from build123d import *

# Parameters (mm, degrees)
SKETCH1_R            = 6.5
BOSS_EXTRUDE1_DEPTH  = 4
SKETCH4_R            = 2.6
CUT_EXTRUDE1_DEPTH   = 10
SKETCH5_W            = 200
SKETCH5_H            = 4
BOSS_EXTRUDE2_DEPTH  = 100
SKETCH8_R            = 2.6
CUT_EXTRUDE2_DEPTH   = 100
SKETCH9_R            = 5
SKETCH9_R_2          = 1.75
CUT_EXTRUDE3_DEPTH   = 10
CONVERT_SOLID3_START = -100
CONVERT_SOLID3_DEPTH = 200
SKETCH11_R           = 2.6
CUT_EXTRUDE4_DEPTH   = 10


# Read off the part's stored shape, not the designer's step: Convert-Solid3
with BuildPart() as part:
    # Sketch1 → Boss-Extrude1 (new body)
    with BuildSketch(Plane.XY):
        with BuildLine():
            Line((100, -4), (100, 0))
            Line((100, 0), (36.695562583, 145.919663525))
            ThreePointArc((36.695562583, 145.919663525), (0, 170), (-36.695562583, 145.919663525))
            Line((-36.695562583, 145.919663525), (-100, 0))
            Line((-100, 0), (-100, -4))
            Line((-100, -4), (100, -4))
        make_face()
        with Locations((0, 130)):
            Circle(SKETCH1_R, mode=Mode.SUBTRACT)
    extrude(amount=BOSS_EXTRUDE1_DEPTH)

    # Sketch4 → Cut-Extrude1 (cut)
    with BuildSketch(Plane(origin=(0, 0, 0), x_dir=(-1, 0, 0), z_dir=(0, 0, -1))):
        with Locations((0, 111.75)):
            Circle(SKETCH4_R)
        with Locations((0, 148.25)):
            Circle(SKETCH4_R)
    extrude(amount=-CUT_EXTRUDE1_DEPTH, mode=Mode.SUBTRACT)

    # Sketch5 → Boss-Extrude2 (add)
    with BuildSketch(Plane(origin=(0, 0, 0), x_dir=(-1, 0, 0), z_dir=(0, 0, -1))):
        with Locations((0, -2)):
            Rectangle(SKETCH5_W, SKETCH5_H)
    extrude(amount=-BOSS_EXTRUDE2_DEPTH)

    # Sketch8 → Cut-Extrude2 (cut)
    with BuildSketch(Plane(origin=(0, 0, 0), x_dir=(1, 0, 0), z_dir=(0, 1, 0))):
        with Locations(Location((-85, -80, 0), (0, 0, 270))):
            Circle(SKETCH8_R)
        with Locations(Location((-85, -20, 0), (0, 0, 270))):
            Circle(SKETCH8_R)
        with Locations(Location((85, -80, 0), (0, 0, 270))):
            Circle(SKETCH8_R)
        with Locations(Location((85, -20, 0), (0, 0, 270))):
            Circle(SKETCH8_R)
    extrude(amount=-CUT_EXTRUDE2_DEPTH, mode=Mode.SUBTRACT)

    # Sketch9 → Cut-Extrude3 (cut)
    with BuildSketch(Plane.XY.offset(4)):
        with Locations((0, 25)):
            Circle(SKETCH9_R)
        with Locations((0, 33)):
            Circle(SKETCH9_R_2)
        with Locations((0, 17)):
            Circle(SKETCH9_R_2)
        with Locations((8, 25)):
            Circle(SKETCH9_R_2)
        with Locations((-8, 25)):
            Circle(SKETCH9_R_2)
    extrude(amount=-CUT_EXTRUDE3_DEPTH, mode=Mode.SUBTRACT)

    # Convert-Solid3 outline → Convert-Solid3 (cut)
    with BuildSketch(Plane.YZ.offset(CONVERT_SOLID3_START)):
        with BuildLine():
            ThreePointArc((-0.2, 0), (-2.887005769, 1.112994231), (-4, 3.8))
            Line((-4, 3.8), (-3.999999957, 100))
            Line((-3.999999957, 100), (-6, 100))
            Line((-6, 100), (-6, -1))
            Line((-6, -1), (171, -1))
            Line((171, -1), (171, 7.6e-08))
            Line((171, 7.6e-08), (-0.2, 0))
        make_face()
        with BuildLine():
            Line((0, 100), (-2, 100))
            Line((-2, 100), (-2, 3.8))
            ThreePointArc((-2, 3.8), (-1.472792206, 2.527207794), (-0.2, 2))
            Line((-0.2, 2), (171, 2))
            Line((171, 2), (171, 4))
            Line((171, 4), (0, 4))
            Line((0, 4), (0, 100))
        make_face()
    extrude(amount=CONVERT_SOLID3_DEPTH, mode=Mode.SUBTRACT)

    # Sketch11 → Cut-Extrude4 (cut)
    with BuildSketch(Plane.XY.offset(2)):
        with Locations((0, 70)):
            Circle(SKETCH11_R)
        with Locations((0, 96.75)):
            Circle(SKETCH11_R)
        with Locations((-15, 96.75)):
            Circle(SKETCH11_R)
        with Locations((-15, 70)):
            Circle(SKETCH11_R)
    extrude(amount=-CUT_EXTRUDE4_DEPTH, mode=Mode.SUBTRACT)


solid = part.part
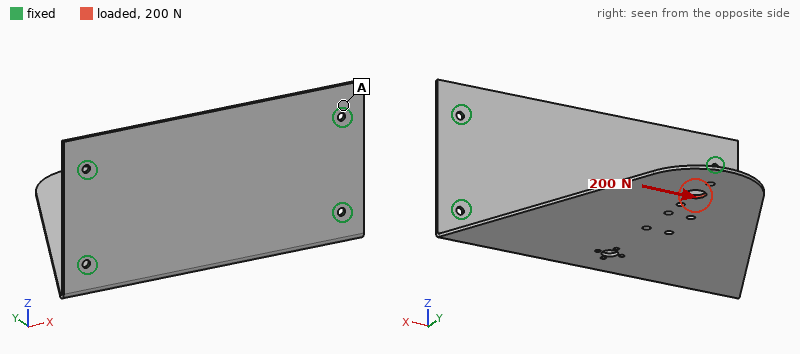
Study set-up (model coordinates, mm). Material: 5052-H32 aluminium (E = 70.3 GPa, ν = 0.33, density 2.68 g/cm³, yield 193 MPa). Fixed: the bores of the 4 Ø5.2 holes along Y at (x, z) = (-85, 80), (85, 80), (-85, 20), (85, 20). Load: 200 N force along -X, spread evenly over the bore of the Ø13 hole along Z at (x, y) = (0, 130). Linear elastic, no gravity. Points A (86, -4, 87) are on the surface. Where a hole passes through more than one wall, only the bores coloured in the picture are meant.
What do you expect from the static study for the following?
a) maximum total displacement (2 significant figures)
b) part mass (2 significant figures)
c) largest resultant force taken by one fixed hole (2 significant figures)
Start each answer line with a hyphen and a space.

- 0.37 mm
- 220 g
- 190 N
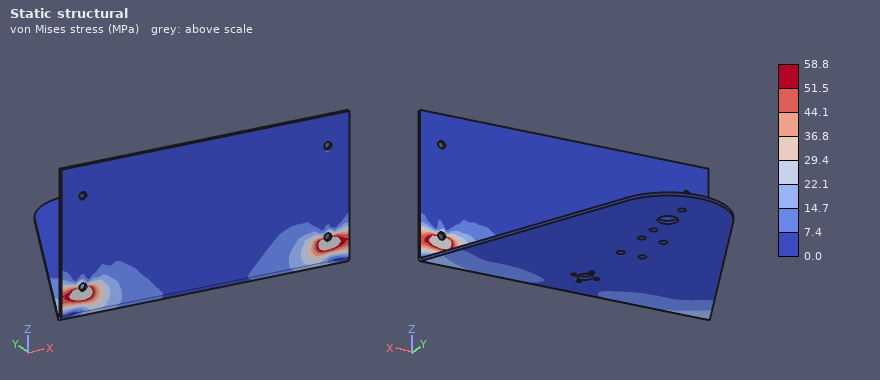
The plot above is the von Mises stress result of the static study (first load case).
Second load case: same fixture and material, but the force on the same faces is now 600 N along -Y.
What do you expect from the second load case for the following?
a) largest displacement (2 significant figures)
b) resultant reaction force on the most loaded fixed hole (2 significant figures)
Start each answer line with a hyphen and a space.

- 2.6 mm
- 360 N
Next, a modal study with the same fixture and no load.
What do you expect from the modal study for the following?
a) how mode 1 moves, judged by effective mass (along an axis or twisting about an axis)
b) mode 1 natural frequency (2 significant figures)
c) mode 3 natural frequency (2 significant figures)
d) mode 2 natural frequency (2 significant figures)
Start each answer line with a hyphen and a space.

- along Z
- 67 Hz
- 330 Hz
- 260 Hz
